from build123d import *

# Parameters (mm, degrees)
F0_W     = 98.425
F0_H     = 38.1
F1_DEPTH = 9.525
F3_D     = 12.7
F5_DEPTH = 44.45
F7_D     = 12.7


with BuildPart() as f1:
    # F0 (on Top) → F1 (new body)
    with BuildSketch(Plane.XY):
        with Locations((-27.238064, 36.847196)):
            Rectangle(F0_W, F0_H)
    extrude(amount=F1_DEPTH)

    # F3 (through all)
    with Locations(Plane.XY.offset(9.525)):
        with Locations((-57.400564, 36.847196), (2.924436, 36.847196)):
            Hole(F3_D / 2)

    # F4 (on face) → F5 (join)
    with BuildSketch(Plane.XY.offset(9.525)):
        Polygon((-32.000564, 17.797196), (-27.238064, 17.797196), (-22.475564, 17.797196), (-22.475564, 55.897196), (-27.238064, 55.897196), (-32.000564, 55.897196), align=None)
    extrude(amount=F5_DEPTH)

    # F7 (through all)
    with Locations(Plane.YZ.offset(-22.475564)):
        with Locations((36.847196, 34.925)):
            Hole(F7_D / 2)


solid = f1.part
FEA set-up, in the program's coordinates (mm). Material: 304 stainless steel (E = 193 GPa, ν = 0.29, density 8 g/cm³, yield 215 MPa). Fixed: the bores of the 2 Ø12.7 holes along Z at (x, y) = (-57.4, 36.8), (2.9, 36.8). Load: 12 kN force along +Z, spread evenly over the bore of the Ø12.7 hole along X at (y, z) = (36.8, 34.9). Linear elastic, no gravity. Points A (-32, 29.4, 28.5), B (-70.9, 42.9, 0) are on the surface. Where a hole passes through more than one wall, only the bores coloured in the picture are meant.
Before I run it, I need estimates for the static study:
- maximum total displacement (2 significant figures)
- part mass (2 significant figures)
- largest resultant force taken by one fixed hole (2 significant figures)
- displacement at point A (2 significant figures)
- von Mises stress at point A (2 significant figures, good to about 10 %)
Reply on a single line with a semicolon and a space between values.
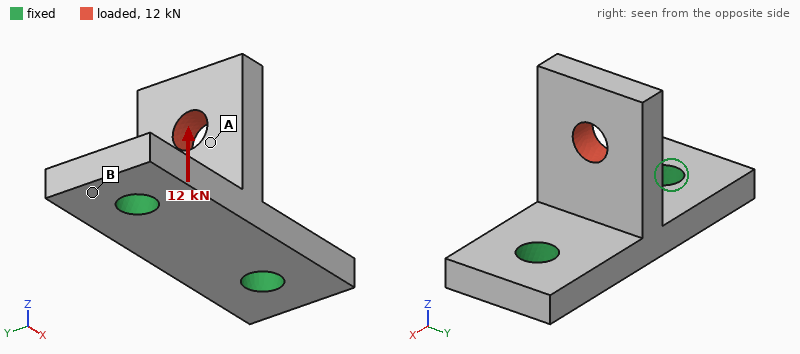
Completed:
30 µm; 390 g; 6.1 kN; 26 µm; 54 MPa
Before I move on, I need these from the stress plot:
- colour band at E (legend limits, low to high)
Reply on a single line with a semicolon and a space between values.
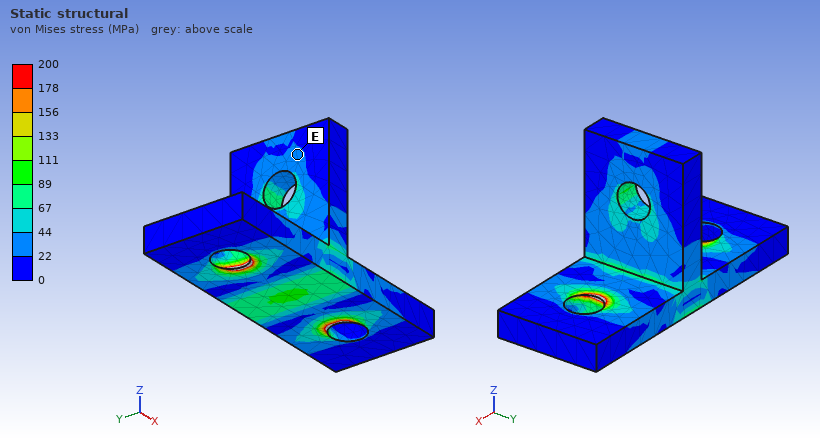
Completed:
22 to 44 MPa
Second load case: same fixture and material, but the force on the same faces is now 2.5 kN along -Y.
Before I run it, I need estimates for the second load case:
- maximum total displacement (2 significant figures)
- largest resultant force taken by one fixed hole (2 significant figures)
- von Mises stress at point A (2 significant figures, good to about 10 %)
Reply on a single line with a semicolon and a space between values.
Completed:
57 µm; 1.3 kN; 12 MPa
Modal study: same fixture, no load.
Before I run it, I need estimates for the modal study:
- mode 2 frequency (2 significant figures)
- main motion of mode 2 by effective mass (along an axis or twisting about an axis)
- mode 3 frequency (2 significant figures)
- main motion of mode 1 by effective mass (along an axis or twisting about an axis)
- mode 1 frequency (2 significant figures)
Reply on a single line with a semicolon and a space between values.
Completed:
3700 Hz; along Y; 7700 Hz; along X; 3000 Hz
